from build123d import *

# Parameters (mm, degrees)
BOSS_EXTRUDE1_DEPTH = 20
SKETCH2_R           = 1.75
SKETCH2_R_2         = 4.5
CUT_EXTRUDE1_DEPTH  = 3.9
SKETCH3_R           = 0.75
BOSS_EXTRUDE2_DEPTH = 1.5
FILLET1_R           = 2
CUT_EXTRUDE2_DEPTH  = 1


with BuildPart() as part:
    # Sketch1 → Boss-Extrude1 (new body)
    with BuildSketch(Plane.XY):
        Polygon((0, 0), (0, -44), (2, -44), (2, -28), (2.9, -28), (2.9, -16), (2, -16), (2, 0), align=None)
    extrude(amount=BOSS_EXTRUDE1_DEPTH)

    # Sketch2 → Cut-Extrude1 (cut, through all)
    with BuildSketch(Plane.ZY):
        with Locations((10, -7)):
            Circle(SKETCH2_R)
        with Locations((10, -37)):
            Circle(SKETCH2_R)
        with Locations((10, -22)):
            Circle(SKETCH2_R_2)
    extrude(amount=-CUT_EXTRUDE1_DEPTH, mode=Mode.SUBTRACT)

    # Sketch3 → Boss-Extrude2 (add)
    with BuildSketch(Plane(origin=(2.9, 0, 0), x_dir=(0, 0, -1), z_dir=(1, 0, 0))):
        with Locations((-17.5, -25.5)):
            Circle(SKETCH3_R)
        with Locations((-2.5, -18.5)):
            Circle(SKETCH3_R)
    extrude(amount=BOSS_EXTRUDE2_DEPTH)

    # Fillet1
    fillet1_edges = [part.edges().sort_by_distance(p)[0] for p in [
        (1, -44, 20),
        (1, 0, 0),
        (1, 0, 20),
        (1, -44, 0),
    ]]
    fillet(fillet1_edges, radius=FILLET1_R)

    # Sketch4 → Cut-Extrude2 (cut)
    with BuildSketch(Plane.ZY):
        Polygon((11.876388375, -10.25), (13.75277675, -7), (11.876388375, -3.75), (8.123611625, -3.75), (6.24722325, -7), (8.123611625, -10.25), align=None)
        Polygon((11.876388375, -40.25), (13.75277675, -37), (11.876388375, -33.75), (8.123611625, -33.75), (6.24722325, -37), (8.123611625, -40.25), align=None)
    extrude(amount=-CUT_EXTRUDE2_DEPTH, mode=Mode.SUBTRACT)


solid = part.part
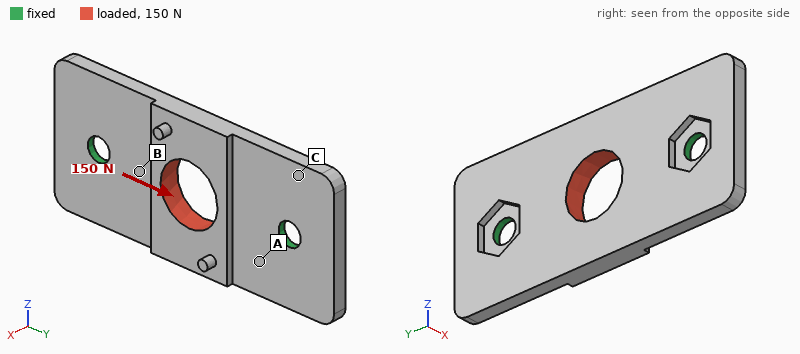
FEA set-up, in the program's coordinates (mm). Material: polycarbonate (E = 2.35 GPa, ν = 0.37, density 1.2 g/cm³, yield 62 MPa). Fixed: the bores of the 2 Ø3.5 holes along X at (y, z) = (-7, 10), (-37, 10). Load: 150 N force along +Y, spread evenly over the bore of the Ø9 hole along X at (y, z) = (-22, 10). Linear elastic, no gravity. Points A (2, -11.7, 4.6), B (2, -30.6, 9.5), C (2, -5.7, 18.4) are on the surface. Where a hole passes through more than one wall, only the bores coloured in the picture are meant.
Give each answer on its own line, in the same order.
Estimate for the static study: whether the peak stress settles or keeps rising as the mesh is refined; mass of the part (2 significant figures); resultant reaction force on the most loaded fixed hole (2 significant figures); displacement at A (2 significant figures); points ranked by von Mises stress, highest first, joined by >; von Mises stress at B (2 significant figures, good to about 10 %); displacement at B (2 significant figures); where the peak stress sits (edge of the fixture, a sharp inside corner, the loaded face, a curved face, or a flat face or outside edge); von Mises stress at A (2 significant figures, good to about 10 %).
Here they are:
keeps rising
2.0 g
75 N
18 µm
B > A > C
6.2 MPa
19 µm
edge of the fixture
3.1 MPa
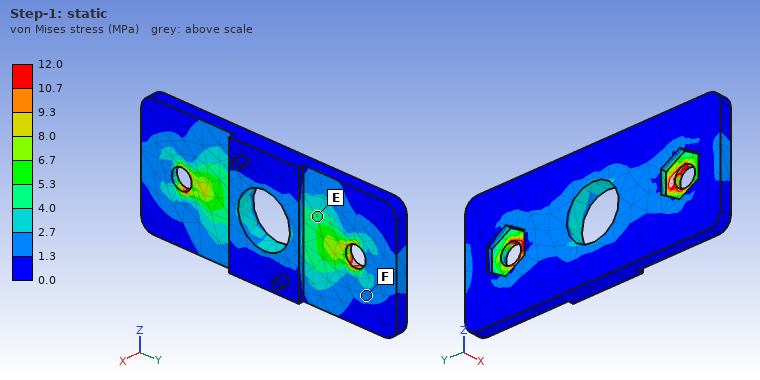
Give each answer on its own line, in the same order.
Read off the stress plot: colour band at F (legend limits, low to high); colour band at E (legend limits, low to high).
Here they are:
1.3 to 2.7 MPa
4.0 to 5.3 MPa
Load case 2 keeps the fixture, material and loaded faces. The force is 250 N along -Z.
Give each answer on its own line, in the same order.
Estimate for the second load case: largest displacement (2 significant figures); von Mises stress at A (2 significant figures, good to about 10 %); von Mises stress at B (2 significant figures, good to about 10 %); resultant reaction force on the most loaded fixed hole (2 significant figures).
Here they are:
0.11 mm
8.8 MPa
9.8 MPa
130 N
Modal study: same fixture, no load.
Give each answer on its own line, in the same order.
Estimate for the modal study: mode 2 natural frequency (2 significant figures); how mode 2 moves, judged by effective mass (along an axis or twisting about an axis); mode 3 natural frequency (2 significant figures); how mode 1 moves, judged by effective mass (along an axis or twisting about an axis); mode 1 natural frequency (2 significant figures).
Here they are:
2300 Hz
along X
3400 Hz
twisting about Y
1800 Hz
